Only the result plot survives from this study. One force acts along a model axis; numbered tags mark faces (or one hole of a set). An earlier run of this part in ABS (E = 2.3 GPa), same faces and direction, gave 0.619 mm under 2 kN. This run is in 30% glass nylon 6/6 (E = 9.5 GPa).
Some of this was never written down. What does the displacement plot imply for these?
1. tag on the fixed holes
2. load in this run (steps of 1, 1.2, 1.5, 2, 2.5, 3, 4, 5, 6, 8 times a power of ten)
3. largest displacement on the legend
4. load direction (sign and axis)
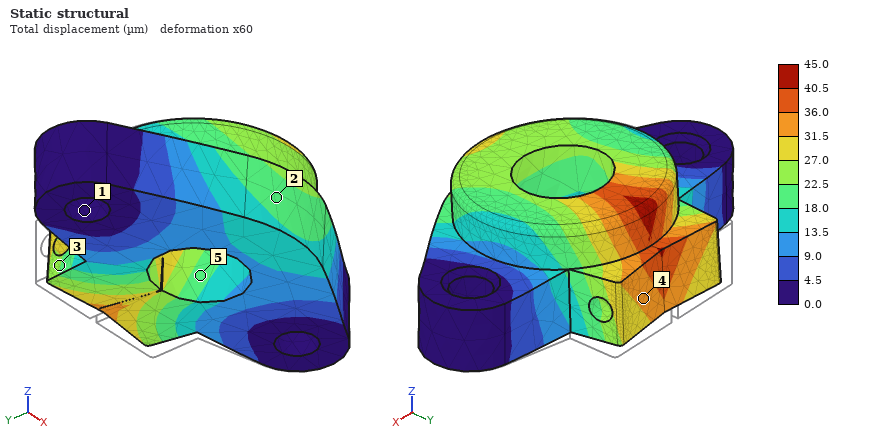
1
600 N
45.0 µm
-Y
